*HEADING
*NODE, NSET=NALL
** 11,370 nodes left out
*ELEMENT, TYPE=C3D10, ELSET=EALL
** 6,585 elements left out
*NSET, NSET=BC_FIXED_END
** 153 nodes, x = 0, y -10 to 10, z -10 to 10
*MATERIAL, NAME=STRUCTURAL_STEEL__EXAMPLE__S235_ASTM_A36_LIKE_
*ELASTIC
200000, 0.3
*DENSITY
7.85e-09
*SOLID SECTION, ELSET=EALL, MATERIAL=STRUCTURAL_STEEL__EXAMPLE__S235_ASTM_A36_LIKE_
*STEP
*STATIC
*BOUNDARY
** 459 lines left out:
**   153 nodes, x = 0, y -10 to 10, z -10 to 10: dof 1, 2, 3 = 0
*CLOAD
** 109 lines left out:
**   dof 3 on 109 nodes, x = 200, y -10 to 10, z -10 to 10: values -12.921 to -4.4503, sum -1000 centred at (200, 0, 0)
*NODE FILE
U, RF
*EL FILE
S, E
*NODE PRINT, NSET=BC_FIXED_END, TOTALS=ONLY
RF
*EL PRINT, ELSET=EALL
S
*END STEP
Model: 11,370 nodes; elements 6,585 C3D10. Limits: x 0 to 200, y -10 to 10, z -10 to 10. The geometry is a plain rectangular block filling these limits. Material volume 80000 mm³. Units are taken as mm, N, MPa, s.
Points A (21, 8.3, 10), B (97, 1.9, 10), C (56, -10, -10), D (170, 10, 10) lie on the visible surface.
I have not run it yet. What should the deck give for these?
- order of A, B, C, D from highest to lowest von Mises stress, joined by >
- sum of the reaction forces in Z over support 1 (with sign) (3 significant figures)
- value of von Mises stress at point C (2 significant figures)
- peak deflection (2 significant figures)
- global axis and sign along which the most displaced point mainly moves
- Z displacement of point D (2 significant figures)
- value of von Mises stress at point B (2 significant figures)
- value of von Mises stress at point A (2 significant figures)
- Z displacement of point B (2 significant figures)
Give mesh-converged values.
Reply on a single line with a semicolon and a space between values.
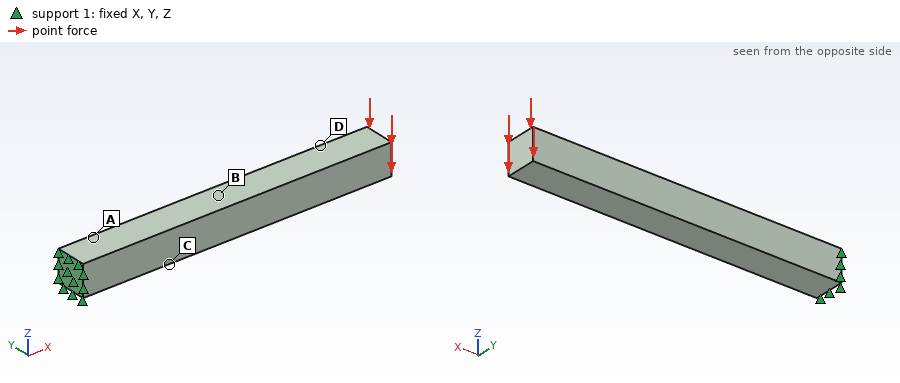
A > C > B > D; 1000 N; 110 MPa; 1.0 mm; -Z; -0.78 mm; 77 MPa; 130 MPa; -0.30 mm
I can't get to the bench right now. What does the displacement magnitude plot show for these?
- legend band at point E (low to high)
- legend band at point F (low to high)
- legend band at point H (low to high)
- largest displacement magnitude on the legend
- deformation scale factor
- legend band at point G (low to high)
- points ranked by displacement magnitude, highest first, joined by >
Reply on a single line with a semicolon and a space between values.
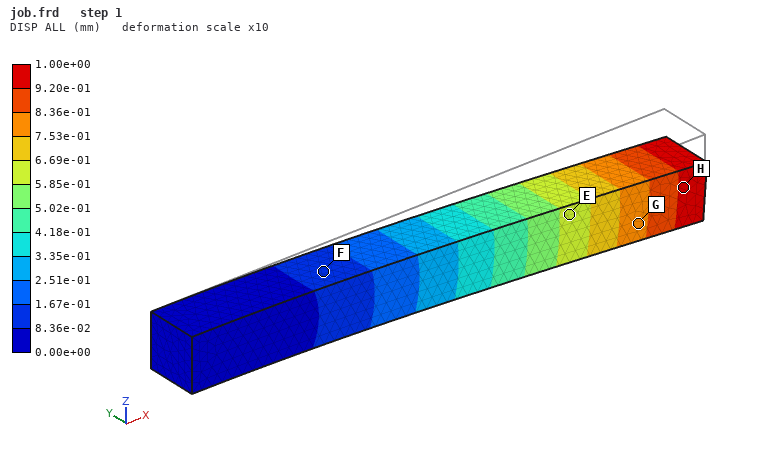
5.85e-01 to 6.69e-01 mm; 8.36e-02 to 1.67e-01 mm; 9.20e-01 to 1.00e+00 mm; 1.00e+00 mm; 10; 7.53e-01 to 8.36e-01 mm; H > G > E > F
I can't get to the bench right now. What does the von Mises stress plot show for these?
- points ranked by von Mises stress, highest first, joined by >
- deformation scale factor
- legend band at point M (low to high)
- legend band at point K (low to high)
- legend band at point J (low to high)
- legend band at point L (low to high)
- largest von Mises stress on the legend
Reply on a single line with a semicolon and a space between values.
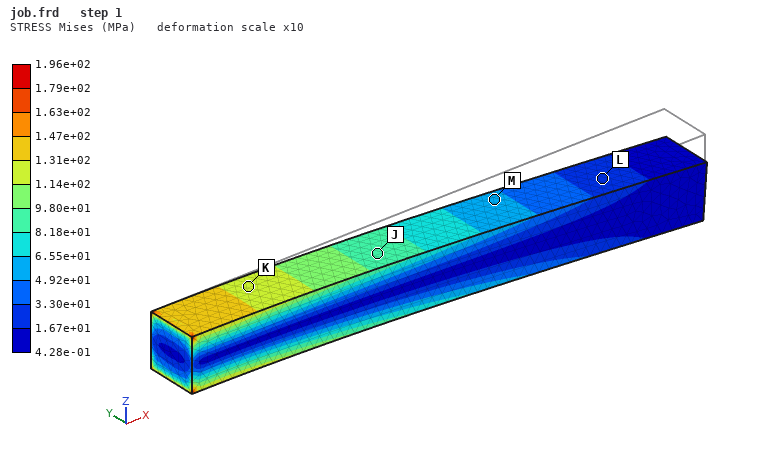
K > J > M > L; 10; 4.92e+01 to 6.55e+01 MPa; 1.14e+02 to 1.31e+02 MPa; 8.18e+01 to 9.80e+01 MPa; 1.67e+01 to 3.30e+01 MPa; 1.96e+02 MPa
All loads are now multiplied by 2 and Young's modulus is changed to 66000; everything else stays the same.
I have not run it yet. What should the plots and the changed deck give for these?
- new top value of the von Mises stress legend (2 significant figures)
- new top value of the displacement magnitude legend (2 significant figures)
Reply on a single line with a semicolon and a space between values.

390 MPa; 6.1 mm
